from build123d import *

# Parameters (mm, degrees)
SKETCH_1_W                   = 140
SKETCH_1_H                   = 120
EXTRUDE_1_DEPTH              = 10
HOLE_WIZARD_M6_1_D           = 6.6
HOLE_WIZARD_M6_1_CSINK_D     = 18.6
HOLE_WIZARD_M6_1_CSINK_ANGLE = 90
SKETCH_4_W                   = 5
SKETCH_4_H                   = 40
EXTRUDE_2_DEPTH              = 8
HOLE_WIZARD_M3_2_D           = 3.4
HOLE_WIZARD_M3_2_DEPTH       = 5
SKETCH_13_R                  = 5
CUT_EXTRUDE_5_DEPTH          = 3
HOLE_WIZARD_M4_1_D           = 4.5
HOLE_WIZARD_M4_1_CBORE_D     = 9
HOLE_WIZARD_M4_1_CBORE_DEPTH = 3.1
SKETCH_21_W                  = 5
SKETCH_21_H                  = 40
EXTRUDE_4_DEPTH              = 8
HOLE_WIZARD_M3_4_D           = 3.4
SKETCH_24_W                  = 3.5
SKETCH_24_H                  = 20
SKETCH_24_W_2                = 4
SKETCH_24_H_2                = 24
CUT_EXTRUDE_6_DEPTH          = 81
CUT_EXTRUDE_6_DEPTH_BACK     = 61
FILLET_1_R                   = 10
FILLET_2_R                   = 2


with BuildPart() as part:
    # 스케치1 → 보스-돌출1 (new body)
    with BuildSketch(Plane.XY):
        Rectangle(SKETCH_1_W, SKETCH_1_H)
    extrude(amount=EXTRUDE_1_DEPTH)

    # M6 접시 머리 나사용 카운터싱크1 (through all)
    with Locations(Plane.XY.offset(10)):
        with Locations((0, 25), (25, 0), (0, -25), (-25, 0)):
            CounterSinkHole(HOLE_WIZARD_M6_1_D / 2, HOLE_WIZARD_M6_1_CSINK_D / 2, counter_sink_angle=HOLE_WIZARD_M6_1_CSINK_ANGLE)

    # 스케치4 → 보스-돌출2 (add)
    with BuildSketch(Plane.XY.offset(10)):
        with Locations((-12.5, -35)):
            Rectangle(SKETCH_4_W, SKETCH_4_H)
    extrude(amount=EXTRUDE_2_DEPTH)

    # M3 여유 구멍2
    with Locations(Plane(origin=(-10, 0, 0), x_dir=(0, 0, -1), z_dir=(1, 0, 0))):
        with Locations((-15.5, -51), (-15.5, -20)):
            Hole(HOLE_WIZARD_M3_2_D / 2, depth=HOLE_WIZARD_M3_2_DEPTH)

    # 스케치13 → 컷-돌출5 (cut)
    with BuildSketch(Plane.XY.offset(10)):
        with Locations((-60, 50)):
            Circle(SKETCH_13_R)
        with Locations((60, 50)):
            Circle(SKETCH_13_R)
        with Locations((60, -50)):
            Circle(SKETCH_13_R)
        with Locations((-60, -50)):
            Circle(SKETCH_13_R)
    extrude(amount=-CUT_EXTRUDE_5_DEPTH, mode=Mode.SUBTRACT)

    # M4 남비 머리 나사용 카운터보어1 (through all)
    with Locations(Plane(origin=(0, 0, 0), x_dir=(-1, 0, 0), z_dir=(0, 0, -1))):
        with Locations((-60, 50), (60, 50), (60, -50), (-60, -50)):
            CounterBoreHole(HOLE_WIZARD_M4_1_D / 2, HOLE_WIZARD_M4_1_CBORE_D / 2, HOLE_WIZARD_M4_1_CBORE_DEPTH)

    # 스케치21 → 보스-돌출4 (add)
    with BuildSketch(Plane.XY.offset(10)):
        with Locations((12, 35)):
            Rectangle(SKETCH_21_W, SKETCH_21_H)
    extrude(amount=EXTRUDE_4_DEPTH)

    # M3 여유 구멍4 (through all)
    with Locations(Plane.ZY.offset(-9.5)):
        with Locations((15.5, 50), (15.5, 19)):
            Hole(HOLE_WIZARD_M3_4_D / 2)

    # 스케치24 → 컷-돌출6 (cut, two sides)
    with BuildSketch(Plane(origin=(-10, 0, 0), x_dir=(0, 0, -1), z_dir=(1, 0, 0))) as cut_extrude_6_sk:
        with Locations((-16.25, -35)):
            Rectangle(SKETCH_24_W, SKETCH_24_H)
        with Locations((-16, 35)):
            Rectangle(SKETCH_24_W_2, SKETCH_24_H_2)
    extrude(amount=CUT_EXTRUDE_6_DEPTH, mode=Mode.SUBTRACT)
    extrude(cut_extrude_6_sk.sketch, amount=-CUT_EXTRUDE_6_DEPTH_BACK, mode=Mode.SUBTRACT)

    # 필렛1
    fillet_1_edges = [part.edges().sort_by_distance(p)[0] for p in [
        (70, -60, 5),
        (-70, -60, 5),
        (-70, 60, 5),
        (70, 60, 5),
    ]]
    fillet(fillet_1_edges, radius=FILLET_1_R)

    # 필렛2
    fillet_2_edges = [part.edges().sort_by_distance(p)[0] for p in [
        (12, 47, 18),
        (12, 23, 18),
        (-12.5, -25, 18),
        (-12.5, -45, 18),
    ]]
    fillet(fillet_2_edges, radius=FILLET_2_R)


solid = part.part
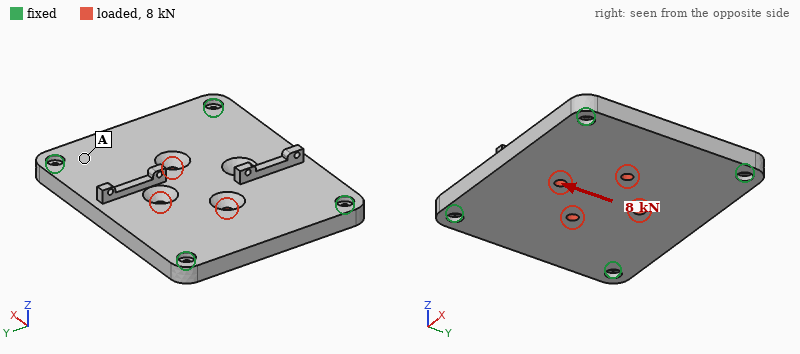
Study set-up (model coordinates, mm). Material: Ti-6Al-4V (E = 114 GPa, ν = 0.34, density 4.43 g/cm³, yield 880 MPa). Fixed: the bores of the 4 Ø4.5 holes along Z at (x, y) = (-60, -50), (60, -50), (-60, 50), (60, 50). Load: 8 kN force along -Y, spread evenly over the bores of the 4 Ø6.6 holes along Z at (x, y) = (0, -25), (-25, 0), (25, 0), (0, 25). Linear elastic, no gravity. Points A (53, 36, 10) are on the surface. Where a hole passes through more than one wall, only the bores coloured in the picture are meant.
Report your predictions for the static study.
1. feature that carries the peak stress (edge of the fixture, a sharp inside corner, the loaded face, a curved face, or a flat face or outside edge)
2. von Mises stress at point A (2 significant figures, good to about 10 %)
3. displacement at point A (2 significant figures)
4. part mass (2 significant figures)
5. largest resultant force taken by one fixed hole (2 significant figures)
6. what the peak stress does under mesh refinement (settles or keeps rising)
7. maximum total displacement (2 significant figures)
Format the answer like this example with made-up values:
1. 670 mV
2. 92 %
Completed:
1. edge of the fixture
2. 6.4 MPa
3. 2.9 µm
4. 720 g
5. 2.2 kN
6. keeps rising
7. 11 µm
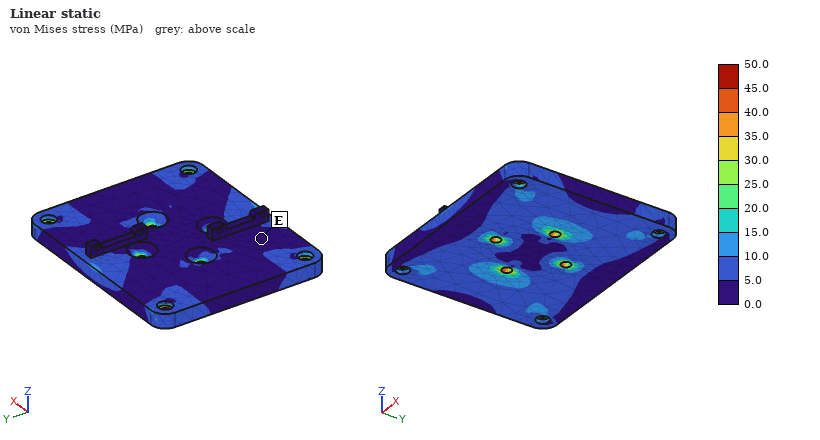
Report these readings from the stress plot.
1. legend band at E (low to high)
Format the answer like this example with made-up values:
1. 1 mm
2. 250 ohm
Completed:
1. 0.0 to 5.0 MPa
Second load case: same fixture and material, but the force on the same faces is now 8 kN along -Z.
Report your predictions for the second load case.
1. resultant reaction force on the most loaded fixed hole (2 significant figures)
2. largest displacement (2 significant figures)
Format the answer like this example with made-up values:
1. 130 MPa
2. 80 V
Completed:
1. 2.1 kN
2. 0.22 mm
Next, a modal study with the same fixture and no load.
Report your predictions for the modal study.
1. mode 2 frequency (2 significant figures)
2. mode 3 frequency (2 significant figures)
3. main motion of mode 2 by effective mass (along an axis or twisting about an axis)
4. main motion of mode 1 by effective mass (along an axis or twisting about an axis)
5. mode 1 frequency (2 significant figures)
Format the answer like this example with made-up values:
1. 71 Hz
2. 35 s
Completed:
1. 3000 Hz
2. 3500 Hz
3. twisting about X
4. along Z
5. 1800 Hz
